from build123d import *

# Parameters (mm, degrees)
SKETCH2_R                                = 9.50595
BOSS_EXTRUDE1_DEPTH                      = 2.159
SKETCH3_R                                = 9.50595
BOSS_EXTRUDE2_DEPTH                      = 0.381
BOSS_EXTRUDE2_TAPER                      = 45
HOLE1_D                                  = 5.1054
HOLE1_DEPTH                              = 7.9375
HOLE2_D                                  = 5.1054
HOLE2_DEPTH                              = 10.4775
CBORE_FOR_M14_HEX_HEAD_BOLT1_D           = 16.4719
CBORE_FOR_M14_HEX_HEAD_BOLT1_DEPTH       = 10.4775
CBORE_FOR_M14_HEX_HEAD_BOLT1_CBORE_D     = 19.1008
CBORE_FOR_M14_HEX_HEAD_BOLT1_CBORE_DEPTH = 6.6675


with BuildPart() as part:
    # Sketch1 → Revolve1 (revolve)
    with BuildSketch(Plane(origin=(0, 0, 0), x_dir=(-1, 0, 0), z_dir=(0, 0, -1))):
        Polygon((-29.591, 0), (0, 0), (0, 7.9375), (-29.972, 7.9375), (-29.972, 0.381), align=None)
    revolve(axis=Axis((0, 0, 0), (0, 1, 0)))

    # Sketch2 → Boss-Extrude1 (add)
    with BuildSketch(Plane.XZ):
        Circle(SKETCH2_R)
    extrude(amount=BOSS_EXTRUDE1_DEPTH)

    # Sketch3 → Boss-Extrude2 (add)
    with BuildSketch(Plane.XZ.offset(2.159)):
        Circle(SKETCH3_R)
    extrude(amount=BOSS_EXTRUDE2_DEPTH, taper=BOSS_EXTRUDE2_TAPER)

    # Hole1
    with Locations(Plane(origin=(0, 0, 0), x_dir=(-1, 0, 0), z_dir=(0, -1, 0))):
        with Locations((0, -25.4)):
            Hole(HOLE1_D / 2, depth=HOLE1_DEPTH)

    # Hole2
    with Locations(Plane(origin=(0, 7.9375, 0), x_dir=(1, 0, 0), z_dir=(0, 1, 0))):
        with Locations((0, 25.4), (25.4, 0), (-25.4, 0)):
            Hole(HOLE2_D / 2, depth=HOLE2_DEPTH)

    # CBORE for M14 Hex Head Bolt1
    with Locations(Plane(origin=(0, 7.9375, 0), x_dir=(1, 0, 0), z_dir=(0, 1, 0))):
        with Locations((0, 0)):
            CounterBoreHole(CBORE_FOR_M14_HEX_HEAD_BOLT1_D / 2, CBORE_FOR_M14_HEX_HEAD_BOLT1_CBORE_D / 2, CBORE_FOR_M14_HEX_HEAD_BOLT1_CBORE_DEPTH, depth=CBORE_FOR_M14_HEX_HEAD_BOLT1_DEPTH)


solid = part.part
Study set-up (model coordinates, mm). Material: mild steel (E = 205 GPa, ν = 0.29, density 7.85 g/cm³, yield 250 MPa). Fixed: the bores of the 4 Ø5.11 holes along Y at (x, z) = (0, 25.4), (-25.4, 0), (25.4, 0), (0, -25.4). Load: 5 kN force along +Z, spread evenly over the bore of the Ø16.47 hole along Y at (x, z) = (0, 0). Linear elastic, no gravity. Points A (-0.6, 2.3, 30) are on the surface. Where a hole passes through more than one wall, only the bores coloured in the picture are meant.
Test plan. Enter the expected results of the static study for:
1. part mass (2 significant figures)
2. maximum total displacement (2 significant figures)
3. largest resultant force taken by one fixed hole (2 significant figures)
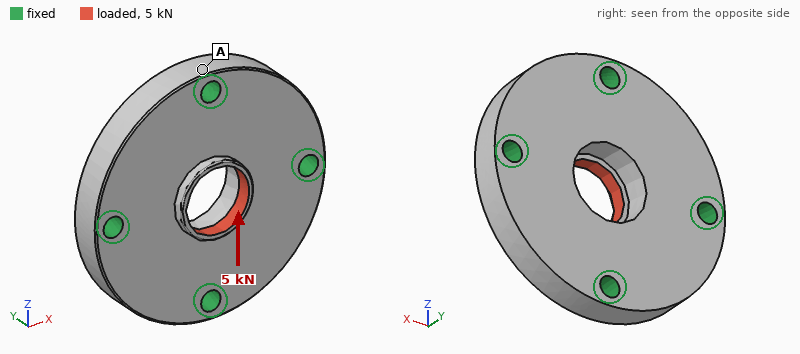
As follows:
150 g
9.1 µm
1.6 kN
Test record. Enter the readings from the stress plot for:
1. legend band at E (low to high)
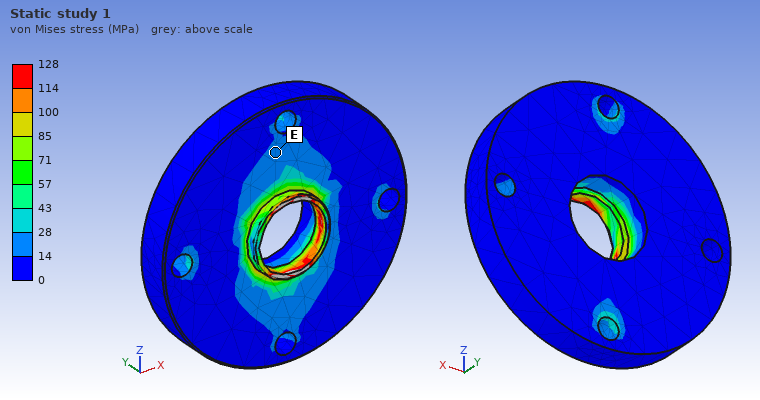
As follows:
14 to 28 MPa
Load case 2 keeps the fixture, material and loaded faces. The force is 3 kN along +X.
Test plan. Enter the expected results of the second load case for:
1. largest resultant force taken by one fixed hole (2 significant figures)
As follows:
970 N
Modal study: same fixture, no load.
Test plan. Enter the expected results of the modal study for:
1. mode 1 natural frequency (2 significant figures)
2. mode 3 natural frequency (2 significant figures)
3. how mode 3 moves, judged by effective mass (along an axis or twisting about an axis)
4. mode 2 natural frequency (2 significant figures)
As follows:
22 kHz
24 kHz
twisting about Z
22 kHz
